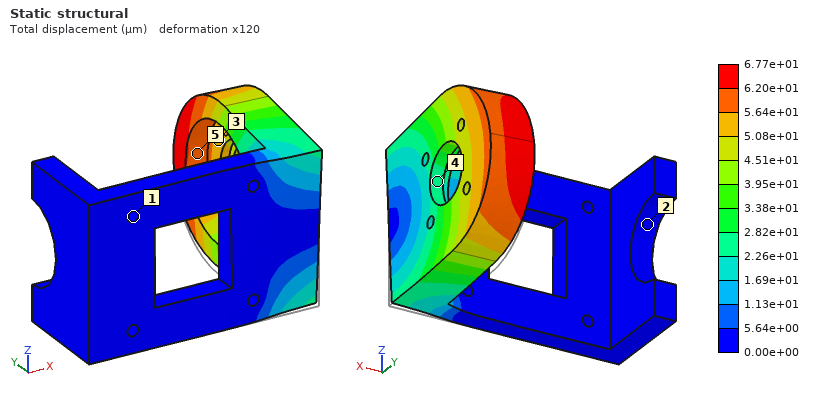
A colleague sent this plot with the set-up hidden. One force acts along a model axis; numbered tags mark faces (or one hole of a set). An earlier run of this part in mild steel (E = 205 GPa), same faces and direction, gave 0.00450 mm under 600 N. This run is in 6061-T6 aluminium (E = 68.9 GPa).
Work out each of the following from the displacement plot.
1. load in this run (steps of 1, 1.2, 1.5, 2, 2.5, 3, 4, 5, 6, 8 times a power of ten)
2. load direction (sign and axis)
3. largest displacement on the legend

3 kN
+Z
6.77e+01 µm
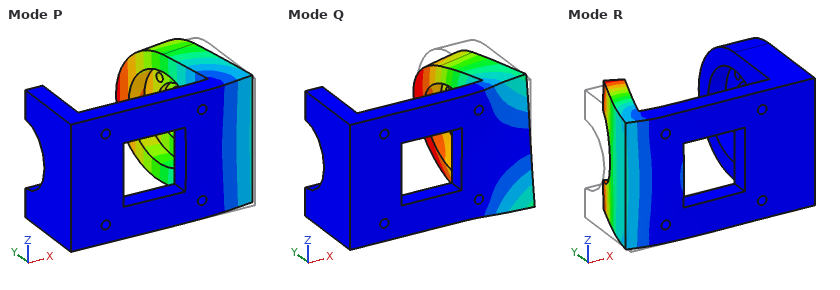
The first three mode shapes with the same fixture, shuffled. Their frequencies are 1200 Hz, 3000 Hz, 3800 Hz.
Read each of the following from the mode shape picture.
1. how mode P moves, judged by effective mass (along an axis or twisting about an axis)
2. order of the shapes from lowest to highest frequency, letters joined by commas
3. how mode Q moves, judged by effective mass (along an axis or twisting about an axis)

along X
P, Q, R
along Z
